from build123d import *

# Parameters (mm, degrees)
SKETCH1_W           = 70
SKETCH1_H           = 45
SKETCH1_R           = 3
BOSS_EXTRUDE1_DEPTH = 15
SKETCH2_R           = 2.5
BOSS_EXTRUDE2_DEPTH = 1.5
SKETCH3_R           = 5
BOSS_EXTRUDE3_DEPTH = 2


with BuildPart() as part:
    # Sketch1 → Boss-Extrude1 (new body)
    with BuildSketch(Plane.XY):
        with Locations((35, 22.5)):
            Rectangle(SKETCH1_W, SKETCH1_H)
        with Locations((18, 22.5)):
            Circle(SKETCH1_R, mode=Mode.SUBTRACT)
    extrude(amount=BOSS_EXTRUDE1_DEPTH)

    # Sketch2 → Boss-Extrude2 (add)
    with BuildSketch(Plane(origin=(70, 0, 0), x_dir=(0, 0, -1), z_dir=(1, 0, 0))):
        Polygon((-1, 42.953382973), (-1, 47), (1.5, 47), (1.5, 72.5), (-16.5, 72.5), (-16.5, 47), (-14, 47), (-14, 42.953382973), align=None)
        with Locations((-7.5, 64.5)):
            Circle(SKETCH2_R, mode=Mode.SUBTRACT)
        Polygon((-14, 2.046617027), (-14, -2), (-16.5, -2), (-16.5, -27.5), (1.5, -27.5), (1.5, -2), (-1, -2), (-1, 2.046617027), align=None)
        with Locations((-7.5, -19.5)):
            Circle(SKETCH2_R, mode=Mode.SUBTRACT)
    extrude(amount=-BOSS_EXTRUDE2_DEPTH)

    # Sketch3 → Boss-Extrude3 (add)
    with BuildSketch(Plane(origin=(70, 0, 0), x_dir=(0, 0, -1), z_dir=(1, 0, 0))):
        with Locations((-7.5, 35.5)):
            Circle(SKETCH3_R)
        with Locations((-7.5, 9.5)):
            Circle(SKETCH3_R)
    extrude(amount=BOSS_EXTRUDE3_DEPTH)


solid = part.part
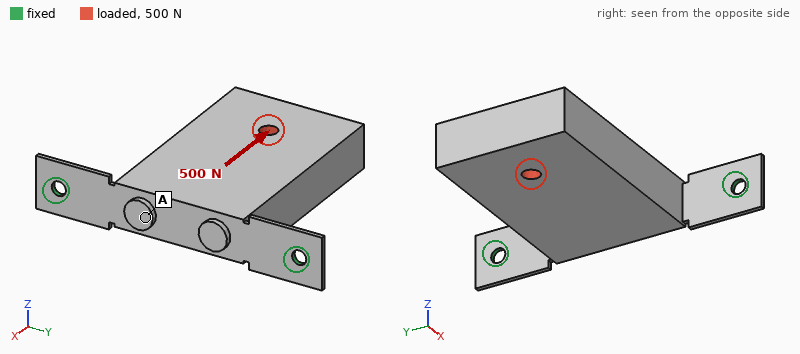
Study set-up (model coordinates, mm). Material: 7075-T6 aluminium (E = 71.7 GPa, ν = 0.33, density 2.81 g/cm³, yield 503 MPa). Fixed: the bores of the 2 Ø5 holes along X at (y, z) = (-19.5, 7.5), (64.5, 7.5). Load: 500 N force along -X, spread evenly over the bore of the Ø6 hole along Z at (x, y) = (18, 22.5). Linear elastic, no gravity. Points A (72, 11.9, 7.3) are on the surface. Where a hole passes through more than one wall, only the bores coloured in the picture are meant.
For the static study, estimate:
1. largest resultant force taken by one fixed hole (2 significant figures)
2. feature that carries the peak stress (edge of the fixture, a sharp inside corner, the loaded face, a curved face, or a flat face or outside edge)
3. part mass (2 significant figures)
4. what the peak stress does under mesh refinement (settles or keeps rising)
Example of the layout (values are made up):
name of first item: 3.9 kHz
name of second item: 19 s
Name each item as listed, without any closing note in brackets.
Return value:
largest resultant force taken by one fixed hole: 310 N
feature that carries the peak stress: edge of the fixture
part mass: 140 g
what the peak stress does under mesh refinement: keeps rising
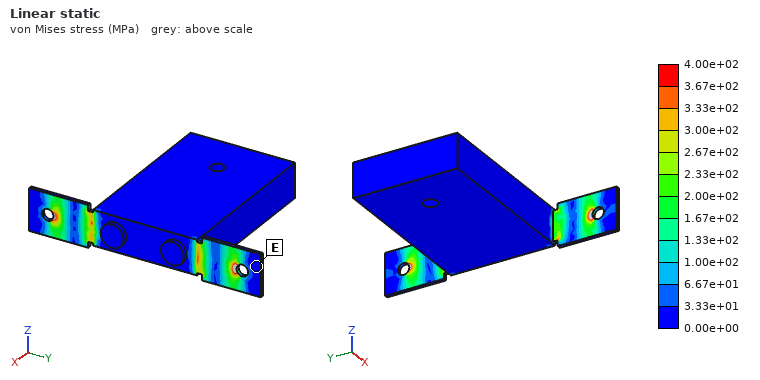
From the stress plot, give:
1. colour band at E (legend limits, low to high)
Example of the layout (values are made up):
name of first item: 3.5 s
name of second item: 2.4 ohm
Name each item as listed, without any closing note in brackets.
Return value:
colour band at E: 0.00e+00 to 3.33e+01 MPa
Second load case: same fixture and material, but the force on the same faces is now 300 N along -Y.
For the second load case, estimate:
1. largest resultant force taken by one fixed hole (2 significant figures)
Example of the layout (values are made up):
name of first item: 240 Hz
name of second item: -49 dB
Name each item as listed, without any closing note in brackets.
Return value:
largest resultant force taken by one fixed hole: 290 N
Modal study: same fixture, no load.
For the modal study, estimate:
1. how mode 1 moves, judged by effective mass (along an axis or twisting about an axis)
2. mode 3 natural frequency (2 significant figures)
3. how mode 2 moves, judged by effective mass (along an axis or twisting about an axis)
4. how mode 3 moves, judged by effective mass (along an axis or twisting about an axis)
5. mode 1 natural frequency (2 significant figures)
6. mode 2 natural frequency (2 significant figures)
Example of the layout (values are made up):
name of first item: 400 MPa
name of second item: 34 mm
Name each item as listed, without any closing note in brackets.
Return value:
how mode 1 moves, judged by effective mass: along Z
mode 3 natural frequency: 470 Hz
how mode 2 moves, judged by effective mass: along Y
how mode 3 moves, judged by effective mass: along X
mode 1 natural frequency: 90 Hz
mode 2 natural frequency: 360 Hz
